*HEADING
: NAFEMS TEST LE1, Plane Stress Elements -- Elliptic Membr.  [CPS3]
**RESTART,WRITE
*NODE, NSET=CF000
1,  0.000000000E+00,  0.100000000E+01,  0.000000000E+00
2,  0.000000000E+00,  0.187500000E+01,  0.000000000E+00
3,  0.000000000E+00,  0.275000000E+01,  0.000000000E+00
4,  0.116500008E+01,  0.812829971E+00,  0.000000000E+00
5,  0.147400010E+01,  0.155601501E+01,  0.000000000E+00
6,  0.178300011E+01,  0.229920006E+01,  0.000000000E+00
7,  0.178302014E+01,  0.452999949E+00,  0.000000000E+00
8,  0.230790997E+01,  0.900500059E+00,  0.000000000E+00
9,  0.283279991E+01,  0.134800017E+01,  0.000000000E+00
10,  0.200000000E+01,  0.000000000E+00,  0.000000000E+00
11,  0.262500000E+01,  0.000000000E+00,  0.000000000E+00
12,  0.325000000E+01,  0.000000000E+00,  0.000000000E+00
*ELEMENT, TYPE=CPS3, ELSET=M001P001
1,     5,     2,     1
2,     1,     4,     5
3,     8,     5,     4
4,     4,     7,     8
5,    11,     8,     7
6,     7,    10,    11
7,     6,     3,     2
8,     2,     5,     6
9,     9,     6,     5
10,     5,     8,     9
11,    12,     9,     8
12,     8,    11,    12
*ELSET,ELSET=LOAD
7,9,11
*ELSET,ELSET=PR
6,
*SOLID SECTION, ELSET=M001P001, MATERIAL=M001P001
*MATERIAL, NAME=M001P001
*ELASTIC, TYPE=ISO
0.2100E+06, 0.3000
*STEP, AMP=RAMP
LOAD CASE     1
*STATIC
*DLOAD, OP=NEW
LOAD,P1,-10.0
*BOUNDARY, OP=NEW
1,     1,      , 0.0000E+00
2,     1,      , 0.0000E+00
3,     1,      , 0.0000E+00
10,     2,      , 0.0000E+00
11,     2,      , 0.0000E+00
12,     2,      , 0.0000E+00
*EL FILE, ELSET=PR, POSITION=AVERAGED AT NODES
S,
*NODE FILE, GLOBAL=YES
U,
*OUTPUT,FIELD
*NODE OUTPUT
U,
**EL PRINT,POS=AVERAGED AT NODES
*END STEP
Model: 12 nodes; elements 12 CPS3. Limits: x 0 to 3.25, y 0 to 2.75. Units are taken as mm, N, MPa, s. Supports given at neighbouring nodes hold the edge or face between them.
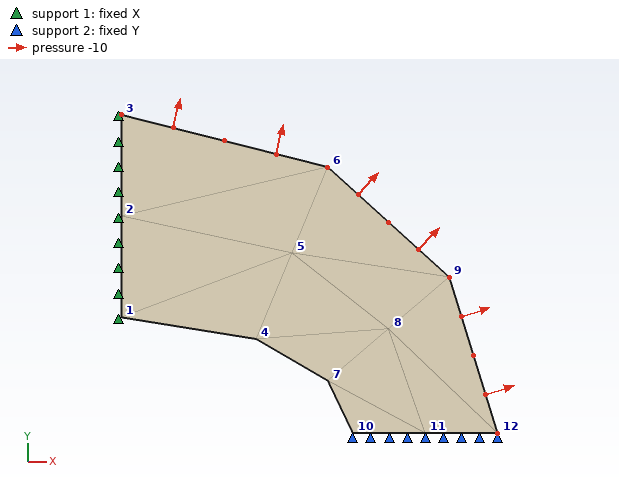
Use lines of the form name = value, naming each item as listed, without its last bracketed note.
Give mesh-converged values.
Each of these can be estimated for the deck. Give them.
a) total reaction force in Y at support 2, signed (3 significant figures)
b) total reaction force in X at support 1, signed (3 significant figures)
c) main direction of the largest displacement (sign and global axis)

total reaction force in Y at support 2, signed = -32.5 N
total reaction force in X at support 1, signed = -27.5 N
main direction of the largest displacement = +Y
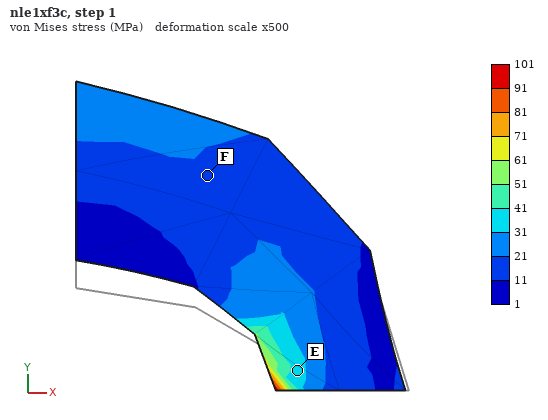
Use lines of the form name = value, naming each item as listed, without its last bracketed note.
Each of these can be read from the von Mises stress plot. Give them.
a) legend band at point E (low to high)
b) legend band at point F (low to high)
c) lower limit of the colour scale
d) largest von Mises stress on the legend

legend band at point E = 31 to 41 MPa
legend band at point F = 11 to 21 MPa
lower limit of the colour scale = 1 MPa
largest von Mises stress on the legend = 101 MPa
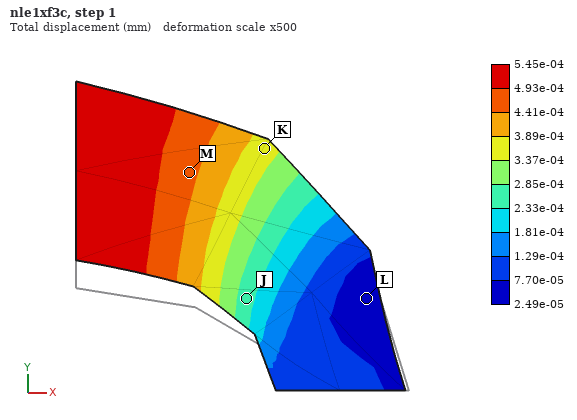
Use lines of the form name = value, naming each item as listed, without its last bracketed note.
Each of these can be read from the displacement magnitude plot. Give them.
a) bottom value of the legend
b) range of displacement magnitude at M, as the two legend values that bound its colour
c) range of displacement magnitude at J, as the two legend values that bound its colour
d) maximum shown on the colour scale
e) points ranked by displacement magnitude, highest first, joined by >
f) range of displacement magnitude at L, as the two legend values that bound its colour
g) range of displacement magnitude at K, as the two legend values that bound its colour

bottom value of the legend = 2.49e-05 mm
range of displacement magnitude at M, as the two legend values that bound its colour = 4.41e-04 to 4.93e-04 mm
range of displacement magnitude at J, as the two legend values that bound its colour = 2.33e-04 to 2.85e-04 mm
maximum shown on the colour scale = 5.45e-04 mm
points ranked by displacement magnitude, highest first, joined by > = M > K > J > L
range of displacement magnitude at L, as the two legend values that bound its colour = 2.49e-05 to 7.70e-05 mm
range of displacement magnitude at K, as the two legend values that bound its colour = 3.37e-04 to 3.89e-04 mm
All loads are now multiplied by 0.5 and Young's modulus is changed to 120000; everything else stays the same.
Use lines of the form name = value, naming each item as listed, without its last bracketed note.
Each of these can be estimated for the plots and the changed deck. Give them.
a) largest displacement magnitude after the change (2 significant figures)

largest displacement magnitude after the change = 4.8e-04 mm
